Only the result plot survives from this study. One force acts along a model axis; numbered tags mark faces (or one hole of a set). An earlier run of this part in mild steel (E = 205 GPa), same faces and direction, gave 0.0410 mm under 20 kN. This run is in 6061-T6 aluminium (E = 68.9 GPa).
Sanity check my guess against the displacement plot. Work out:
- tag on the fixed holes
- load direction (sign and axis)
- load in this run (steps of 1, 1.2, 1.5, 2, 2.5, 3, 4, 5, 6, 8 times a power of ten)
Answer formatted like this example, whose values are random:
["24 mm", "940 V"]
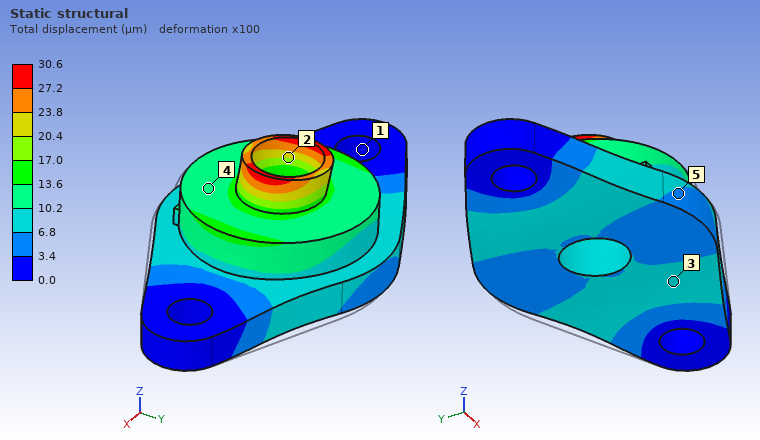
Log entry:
["1", "-X", "5 kN"]
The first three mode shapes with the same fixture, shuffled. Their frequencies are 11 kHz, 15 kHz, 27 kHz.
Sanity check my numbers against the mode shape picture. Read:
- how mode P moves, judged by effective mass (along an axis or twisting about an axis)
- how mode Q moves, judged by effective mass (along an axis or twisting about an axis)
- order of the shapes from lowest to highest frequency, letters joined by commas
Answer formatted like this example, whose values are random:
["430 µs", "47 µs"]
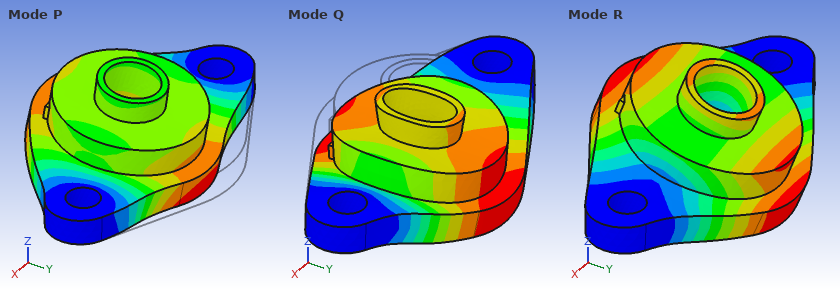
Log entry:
["along Y", "along Z", "R, Q, P"]
